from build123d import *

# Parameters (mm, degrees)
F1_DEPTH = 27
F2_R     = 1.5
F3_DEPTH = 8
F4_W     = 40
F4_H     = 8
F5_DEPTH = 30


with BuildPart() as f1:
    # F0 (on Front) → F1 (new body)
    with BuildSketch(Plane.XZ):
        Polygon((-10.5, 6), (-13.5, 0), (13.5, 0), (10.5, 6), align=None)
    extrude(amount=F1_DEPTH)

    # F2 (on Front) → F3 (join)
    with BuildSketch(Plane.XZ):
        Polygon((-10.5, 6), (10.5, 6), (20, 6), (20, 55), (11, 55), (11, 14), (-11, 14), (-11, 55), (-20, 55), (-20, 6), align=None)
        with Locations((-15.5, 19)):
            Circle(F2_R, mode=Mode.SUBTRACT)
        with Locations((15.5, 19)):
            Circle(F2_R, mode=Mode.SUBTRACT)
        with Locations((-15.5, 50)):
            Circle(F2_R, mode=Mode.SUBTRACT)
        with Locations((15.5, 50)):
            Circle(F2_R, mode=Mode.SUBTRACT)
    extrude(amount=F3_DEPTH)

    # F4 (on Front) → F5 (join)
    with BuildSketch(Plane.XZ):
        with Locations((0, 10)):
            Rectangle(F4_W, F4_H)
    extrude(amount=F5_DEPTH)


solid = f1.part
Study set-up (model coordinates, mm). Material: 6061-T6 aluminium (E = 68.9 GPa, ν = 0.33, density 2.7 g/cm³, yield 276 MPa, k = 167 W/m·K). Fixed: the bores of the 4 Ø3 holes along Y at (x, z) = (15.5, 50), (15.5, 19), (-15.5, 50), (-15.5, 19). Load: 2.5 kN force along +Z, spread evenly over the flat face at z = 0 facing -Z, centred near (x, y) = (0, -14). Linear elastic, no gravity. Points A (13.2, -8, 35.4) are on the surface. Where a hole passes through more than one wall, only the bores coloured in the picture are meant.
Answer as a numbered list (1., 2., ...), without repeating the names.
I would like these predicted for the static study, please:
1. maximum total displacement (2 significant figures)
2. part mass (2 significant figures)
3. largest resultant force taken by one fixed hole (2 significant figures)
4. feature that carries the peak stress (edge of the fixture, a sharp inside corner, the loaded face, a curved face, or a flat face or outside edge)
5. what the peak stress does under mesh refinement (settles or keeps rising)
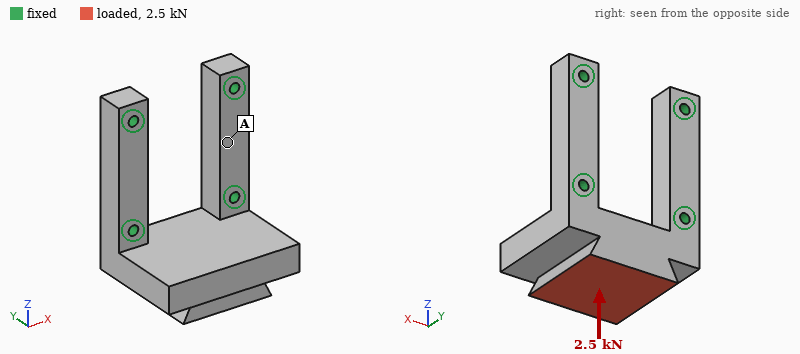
1. 0.12 mm
2. 52 g
3. 1.3 kN
4. edge of the fixture
5. keeps rising
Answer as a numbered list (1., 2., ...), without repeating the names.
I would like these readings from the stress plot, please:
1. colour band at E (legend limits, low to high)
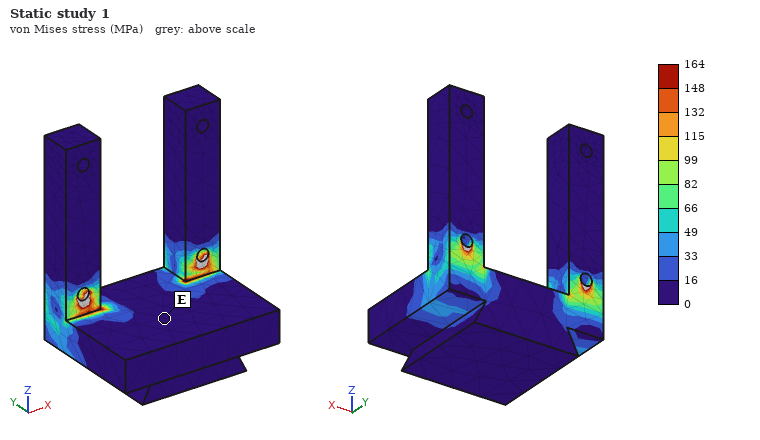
1. 0 to 16 MPa
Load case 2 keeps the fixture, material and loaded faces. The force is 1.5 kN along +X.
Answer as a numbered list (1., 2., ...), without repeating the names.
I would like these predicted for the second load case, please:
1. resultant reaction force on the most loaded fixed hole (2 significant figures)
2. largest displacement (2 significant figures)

1. 1.2 kN
2. 13 µm
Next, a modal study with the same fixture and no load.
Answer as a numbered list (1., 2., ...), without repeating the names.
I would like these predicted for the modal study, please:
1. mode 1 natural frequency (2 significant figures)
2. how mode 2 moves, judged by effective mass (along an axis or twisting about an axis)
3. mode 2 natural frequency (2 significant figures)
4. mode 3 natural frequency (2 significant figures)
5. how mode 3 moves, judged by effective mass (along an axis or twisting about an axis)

1. 4000 Hz
2. along X
3. 10 kHz
4. 15 kHz
5. along Y
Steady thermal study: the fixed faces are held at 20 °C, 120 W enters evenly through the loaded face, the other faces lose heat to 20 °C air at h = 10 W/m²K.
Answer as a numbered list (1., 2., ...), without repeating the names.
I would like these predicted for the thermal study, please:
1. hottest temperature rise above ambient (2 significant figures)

1. 68 K
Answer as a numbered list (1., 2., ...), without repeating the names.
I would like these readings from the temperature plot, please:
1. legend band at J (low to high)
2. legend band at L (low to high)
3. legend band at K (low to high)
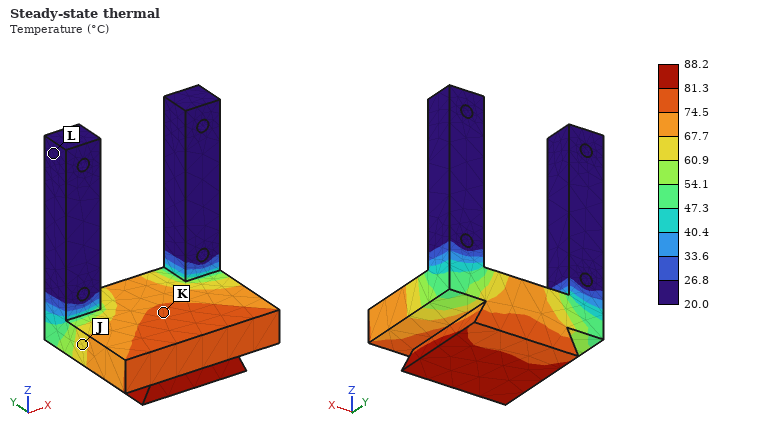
1. 60.9 to 67.7 °C
2. 20.0 to 26.8 °C
3. 74.5 to 81.3 °C
